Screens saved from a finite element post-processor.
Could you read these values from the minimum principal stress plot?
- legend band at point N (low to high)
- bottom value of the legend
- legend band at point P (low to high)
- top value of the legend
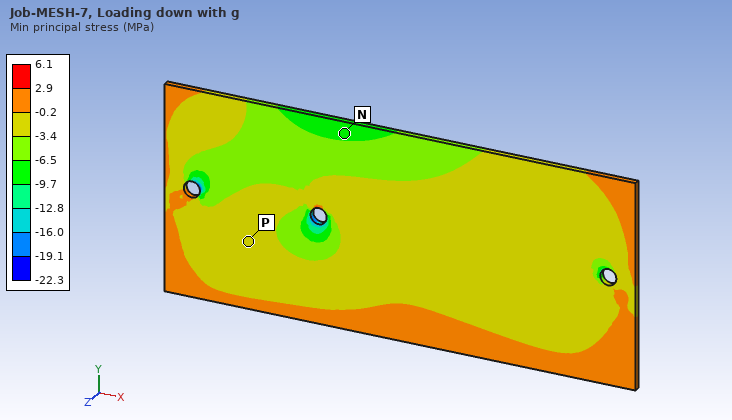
-9.7 to -6.5 MPa
-22.3 MPa
-3.4 to -0.2 MPa
6.1 MPa
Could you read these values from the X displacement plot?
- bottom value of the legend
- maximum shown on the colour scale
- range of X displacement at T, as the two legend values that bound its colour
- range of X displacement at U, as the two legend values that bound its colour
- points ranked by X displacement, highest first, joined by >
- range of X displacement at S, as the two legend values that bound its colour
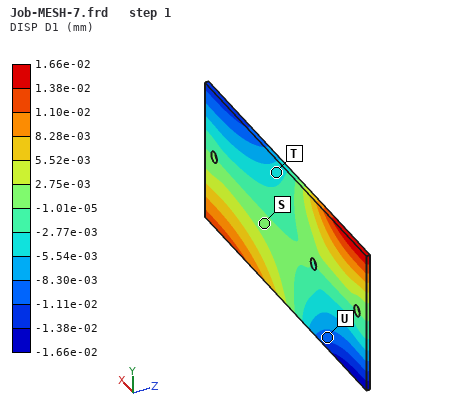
-1.66e-02 mm
1.66e-02 mm
-5.54e-03 to -2.77e-03 mm
-1.11e-02 to -8.30e-03 mm
S > T > U
-1.01e-05 to 2.75e-03 mm
